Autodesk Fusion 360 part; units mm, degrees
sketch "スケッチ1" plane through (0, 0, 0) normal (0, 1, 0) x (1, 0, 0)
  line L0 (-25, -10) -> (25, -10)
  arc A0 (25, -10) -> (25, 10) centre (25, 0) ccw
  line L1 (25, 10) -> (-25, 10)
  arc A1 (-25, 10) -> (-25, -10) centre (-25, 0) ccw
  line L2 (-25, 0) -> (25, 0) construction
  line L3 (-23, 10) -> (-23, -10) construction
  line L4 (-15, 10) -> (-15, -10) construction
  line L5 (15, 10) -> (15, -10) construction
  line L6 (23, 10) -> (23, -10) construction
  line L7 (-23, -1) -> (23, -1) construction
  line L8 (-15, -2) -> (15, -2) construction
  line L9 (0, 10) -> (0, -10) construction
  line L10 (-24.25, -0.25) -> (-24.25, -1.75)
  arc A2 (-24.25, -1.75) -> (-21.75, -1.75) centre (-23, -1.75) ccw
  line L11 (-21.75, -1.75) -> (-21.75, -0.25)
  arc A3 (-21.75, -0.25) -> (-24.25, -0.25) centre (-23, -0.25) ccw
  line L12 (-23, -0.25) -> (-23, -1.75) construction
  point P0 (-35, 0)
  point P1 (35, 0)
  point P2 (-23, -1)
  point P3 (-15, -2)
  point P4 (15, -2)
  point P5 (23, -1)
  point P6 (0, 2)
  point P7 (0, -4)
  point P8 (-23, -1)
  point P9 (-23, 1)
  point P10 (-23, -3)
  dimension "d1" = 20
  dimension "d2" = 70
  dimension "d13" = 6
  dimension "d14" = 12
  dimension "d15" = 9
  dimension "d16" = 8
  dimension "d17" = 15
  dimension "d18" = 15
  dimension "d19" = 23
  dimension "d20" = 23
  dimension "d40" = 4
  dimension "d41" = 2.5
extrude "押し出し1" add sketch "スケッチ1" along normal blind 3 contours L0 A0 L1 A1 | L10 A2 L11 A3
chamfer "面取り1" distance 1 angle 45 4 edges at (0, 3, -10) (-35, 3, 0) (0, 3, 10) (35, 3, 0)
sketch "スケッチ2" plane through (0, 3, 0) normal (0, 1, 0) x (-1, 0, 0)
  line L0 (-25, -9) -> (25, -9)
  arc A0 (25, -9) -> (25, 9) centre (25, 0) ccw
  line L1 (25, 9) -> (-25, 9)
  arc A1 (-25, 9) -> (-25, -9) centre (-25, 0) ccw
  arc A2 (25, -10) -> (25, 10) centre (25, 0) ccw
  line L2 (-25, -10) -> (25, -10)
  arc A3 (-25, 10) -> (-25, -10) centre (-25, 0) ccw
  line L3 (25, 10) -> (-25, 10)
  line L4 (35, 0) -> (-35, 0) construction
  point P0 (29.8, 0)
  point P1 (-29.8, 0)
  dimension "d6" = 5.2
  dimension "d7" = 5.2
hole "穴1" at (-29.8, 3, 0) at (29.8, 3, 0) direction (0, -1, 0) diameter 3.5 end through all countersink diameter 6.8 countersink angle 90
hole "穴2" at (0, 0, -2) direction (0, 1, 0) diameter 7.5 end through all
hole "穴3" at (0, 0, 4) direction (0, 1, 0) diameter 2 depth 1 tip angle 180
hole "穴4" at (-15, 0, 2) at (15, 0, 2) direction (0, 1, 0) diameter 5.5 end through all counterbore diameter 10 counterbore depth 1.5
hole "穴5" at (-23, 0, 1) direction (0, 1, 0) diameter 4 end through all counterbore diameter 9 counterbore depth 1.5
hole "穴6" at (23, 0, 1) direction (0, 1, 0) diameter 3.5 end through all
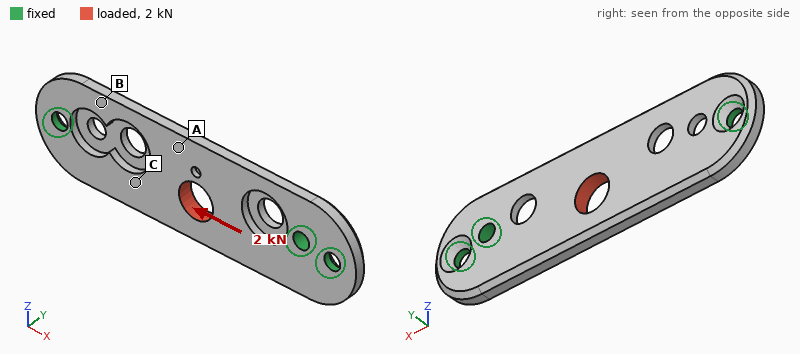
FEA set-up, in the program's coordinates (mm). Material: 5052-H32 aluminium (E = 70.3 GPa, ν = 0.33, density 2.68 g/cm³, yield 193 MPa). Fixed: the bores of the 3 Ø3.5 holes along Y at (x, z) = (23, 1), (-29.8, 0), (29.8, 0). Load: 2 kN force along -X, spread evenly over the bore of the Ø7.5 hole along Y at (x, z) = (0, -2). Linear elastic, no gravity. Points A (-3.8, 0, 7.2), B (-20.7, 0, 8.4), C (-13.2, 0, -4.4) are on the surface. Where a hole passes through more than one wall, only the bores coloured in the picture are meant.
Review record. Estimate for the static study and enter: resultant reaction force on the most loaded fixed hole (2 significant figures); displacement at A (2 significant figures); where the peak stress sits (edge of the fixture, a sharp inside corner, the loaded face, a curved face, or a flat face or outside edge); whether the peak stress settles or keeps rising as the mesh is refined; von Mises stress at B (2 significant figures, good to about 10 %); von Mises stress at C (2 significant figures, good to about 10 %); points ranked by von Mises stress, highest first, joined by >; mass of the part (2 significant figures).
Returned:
840 N
16 µm
edge of the fixture
keeps rising
21 MPa
31 MPa
C > B > A
8.5 g
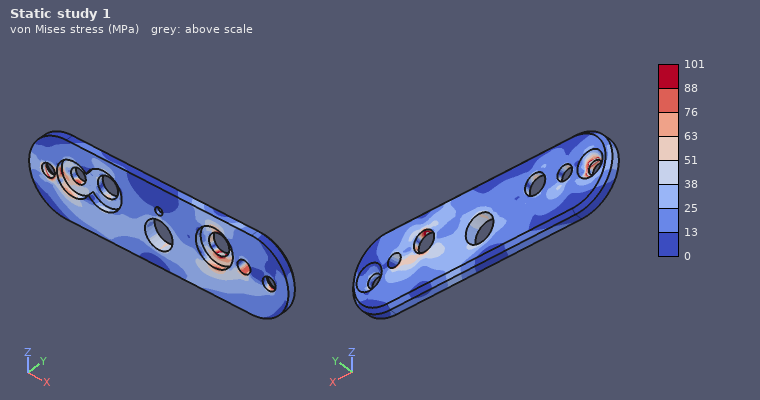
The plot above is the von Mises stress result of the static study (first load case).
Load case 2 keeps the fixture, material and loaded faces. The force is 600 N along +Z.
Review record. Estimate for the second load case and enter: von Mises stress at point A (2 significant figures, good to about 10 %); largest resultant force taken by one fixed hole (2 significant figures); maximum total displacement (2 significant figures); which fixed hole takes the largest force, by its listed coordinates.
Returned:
16 MPa
650 N
23 µm
(23, 1)
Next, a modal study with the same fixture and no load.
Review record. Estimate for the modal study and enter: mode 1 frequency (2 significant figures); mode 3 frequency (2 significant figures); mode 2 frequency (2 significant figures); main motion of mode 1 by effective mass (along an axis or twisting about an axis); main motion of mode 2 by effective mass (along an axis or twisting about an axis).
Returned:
4400 Hz
12 kHz
6900 Hz
along Y
twisting about X
